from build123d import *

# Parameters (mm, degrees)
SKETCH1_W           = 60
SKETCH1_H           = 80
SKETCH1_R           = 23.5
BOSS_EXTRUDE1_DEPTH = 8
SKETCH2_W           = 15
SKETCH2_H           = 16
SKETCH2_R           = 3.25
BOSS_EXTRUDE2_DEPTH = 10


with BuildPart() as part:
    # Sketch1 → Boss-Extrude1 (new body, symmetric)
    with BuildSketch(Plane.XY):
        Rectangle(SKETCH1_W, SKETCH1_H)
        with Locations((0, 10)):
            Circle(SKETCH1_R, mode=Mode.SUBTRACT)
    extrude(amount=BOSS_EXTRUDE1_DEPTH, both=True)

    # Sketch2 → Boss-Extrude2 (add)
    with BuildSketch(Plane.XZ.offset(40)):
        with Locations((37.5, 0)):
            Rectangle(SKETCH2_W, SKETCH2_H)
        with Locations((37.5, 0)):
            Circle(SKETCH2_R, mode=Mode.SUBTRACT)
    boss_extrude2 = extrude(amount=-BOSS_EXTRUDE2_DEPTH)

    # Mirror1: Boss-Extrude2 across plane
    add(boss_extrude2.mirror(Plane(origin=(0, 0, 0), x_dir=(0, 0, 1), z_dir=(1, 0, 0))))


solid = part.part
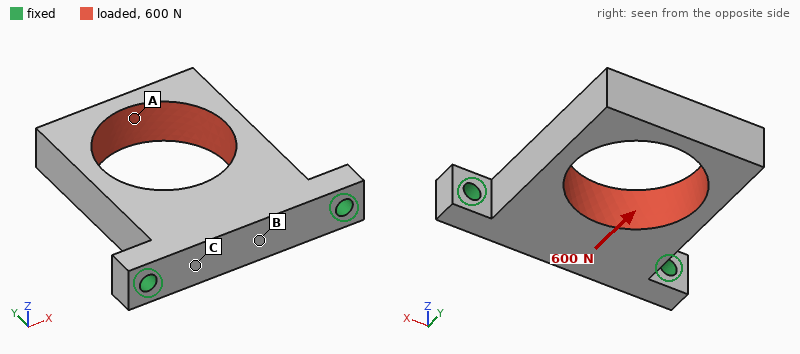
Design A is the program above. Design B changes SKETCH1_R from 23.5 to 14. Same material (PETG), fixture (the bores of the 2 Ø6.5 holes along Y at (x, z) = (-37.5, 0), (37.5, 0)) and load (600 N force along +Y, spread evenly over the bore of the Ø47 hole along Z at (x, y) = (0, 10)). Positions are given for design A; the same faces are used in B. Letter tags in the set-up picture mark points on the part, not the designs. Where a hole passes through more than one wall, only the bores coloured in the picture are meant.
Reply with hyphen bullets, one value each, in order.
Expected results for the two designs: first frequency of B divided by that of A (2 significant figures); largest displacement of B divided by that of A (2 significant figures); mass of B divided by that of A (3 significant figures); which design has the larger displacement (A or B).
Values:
- 0.86
- 0.43
- 1.34
- A
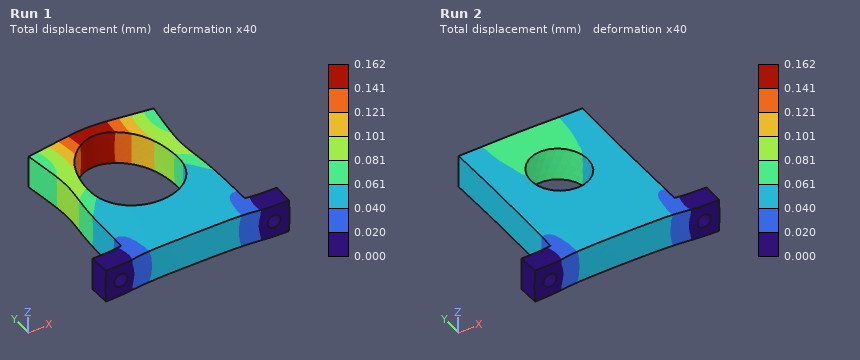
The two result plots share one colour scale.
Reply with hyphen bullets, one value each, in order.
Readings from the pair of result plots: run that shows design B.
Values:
- Run 2
